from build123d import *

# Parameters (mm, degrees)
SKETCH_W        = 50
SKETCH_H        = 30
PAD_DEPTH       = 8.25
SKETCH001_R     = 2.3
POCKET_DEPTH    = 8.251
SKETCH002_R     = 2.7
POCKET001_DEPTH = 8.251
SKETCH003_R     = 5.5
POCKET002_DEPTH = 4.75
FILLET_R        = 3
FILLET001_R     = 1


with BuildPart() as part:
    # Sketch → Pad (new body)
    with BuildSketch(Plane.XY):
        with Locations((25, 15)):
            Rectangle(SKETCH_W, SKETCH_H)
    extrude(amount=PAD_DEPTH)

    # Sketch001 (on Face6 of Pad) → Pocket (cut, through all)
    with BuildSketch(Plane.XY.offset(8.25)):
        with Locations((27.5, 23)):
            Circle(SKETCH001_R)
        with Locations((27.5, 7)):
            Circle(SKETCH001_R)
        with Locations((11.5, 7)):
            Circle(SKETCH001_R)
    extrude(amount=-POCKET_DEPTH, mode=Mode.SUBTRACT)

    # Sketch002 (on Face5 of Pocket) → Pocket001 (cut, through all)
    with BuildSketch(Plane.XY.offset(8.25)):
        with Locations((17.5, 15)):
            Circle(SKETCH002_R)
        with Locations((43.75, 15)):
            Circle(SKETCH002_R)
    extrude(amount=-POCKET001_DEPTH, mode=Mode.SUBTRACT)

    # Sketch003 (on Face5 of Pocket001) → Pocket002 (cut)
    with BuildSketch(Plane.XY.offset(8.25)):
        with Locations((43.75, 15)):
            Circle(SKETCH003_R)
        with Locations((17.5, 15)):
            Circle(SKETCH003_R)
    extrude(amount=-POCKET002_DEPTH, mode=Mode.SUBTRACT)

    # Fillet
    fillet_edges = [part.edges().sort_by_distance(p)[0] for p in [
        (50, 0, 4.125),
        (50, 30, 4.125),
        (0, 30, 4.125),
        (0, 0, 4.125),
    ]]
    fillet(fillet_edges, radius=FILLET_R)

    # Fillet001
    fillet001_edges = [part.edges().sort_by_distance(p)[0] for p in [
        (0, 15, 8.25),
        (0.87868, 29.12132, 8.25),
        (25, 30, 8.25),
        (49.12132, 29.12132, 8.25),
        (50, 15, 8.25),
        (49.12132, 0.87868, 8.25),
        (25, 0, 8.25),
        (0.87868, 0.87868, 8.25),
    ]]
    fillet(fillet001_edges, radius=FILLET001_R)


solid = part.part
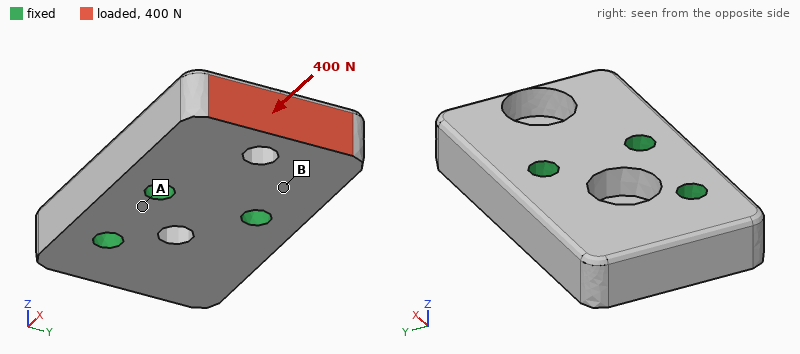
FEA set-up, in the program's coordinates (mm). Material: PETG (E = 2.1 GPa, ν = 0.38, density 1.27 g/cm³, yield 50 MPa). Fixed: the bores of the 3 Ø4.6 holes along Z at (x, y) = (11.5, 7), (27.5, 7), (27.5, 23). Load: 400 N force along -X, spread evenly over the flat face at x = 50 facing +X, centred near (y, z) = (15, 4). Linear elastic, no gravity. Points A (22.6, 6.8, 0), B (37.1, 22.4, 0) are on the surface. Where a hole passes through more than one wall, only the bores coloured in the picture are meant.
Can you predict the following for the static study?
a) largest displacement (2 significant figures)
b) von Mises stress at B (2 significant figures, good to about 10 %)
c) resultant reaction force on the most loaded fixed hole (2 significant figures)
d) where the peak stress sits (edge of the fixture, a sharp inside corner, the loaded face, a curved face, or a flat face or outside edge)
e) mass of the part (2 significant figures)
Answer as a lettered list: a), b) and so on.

a) 90 µm
b) 3.1 MPa
c) 200 N
d) the loaded face
e) 14 g
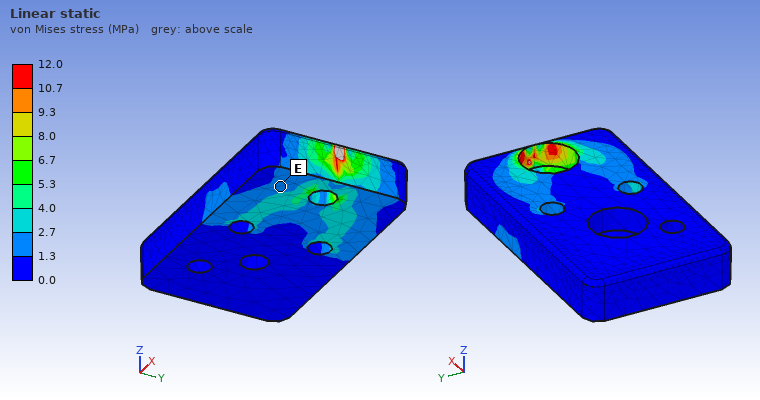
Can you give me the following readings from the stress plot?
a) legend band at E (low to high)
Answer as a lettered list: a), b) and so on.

a) 1.3 to 2.7 MPa
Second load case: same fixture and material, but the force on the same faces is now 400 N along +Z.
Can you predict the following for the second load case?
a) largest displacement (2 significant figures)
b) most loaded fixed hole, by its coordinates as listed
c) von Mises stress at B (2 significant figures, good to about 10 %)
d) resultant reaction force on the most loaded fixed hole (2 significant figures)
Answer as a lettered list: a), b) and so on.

a) 0.70 mm
b) (27.5, 7)
c) 18 MPa
d) 240 N
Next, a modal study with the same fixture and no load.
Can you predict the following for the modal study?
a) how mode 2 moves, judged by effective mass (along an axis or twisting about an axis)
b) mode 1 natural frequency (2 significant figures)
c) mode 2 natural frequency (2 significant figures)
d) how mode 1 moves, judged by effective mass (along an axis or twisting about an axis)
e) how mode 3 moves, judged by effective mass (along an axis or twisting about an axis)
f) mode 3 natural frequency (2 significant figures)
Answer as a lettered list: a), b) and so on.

a) along Z
b) 3500 Hz
c) 4100 Hz
d) along Z
e) twisting about X
f) 5000 Hz
